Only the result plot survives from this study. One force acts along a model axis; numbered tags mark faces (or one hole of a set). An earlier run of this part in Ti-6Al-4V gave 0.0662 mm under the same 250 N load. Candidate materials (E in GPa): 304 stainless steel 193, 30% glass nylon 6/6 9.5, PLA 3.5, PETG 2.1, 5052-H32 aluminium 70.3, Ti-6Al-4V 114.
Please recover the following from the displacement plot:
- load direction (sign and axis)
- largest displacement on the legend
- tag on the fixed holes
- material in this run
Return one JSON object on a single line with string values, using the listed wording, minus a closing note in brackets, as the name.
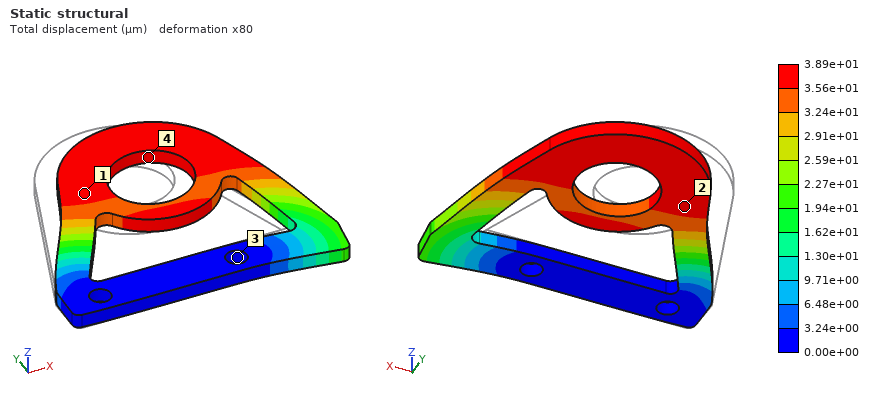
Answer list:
{"load direction": "+X", "largest displacement on the legend": "3.89e+01 µm", "tag on the fixed holes": "3", "material in this run": "304 stainless steel"}
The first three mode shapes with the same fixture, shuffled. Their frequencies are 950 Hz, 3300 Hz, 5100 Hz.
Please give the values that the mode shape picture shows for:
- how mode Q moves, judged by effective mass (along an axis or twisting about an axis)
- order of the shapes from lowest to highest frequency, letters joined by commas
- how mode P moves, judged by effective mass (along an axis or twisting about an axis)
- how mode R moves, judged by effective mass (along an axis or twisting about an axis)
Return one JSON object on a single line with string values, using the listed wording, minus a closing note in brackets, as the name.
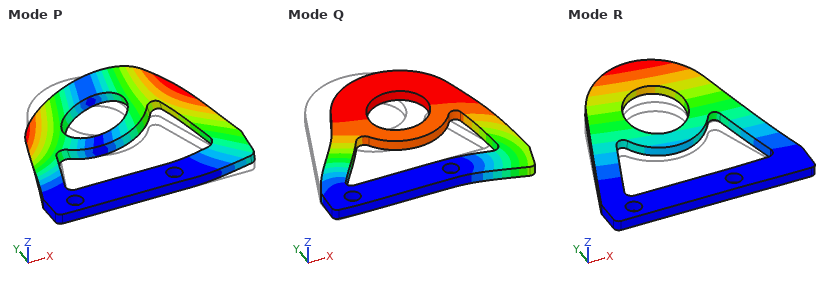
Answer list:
{"how mode Q moves, judged by effective mass": "along X", "order of the shapes from lowest to highest frequency, letters joined by commas": "R, P, Q", "how mode P moves, judged by effective mass": "twisting about Y", "how mode R moves, judged by effective mass": "along Z"}
